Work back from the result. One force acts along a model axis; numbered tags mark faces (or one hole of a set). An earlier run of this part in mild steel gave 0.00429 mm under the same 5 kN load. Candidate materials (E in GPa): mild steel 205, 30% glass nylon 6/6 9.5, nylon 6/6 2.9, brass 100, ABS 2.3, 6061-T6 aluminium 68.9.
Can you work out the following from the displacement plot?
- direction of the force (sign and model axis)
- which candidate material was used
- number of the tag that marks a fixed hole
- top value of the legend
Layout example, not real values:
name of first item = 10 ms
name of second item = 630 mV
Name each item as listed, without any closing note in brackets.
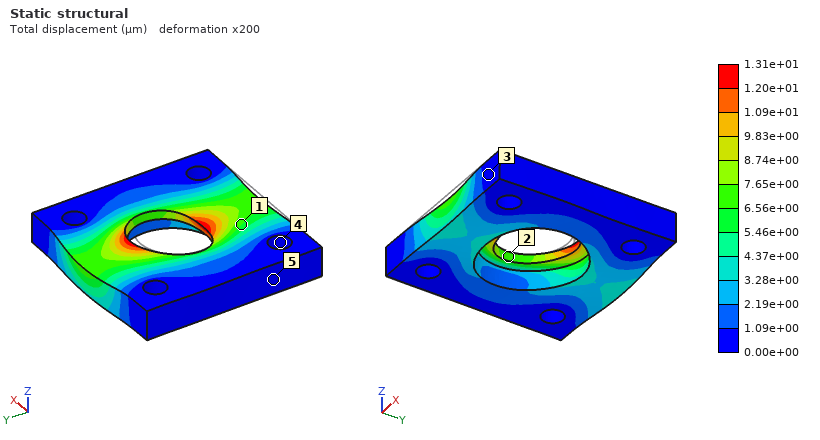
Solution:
direction of the force = +Y
which candidate material was used = 6061-T6 aluminium
number of the tag that marks a fixed hole = 4
top value of the legend = 1.31e+01 µm
